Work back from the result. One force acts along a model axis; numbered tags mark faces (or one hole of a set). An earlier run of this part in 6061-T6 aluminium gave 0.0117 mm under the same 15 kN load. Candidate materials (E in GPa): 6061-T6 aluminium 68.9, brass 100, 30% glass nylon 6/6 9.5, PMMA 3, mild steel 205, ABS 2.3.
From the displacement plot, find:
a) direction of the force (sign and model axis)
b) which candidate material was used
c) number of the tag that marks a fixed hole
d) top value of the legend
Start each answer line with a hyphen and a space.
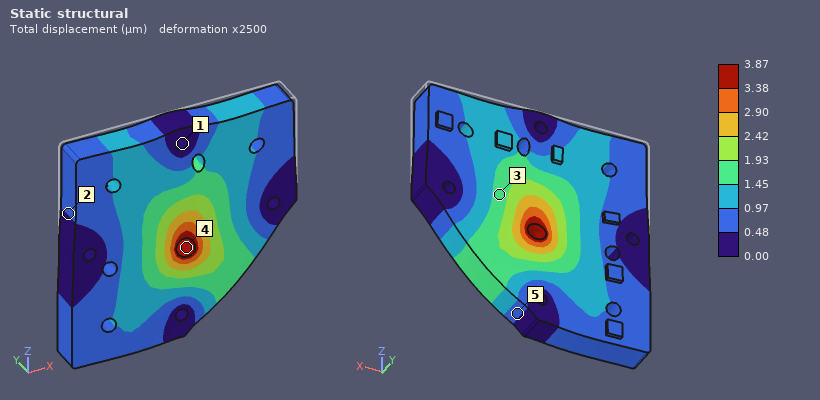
- -Z
- mild steel
- 1
- 3.87 µm
